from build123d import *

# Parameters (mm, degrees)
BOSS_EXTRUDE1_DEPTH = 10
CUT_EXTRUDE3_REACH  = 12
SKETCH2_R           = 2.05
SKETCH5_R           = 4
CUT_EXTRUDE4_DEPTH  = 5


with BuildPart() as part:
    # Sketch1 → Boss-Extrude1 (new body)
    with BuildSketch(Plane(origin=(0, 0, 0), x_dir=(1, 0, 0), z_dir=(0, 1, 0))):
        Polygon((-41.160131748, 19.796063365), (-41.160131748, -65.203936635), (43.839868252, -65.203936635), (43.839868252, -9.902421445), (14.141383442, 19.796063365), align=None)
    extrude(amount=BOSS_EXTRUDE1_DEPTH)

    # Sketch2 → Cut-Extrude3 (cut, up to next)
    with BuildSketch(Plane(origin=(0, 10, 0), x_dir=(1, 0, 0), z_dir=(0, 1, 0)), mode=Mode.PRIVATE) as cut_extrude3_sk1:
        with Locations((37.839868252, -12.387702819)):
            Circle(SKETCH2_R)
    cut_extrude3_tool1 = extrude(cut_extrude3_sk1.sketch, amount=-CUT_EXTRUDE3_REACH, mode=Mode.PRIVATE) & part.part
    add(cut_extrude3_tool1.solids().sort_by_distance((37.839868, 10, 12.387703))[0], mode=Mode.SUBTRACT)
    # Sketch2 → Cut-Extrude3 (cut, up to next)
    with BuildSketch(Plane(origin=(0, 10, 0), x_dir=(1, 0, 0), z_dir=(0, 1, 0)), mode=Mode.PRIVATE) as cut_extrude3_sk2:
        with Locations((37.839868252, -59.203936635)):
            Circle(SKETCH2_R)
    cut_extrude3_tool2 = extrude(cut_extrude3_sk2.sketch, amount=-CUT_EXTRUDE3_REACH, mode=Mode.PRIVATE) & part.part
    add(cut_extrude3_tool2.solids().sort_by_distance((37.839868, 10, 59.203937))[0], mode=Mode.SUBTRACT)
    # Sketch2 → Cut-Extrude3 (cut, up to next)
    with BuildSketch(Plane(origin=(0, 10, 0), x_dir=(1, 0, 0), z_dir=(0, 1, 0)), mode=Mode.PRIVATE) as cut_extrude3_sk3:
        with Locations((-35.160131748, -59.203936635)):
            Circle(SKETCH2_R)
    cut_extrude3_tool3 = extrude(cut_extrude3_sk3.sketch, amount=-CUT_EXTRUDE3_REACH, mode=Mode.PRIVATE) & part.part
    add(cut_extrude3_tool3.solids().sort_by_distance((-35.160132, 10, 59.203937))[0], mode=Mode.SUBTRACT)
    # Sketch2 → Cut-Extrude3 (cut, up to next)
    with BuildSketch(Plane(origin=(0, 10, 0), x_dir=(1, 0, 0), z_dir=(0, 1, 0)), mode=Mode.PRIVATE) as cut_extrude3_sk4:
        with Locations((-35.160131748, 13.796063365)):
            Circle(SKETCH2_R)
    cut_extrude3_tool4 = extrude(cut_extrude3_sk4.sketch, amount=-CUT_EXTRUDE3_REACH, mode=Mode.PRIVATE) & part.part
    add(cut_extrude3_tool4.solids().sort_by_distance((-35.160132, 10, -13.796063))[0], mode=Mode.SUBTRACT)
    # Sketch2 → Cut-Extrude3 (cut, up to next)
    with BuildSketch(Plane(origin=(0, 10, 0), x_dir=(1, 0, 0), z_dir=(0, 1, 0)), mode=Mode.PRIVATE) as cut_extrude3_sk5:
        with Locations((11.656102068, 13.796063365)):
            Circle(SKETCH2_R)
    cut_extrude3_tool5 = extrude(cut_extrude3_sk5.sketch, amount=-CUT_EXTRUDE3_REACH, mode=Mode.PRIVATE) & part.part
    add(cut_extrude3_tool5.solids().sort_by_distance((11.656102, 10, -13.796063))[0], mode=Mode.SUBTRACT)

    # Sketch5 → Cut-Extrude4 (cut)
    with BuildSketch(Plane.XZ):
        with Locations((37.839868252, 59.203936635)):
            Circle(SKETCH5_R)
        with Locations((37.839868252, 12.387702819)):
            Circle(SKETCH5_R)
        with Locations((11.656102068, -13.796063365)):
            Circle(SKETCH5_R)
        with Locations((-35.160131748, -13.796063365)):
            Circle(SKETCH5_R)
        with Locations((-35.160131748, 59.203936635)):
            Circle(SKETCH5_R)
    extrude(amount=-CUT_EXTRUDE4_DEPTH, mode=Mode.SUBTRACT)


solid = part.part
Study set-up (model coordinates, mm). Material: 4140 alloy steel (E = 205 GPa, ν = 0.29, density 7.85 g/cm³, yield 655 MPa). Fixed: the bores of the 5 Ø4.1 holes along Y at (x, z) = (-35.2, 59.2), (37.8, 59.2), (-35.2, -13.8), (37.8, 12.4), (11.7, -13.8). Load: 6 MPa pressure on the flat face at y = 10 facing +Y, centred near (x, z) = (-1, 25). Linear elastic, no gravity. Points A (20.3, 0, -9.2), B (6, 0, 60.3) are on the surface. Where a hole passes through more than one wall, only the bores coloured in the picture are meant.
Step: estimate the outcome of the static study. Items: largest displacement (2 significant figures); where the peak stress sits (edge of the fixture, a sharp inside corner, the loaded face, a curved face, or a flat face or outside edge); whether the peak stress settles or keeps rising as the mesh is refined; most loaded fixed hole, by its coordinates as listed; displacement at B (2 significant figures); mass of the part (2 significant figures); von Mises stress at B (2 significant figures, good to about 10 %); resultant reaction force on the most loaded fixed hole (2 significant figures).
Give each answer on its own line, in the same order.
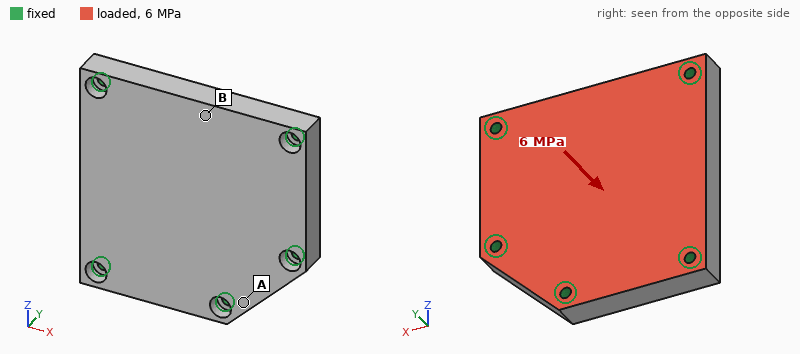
87 µm
edge of the fixture
keeps rising
(-35.2, 59.2)
70 µm
520 g
150 MPa
14 kN
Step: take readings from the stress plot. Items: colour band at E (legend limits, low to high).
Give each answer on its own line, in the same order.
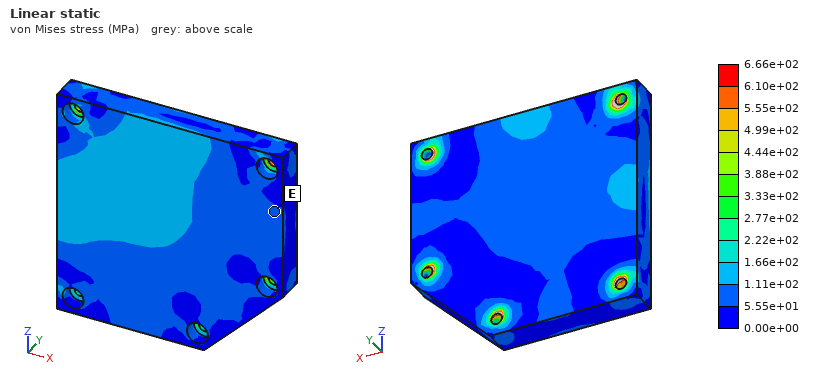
5.55e+01 to 1.11e+02 MPa
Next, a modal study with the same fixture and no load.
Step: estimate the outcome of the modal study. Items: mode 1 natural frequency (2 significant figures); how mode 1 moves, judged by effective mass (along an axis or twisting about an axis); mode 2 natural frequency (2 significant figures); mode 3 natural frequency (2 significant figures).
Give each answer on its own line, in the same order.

5500 Hz
along Y
8100 Hz
12 kHz
